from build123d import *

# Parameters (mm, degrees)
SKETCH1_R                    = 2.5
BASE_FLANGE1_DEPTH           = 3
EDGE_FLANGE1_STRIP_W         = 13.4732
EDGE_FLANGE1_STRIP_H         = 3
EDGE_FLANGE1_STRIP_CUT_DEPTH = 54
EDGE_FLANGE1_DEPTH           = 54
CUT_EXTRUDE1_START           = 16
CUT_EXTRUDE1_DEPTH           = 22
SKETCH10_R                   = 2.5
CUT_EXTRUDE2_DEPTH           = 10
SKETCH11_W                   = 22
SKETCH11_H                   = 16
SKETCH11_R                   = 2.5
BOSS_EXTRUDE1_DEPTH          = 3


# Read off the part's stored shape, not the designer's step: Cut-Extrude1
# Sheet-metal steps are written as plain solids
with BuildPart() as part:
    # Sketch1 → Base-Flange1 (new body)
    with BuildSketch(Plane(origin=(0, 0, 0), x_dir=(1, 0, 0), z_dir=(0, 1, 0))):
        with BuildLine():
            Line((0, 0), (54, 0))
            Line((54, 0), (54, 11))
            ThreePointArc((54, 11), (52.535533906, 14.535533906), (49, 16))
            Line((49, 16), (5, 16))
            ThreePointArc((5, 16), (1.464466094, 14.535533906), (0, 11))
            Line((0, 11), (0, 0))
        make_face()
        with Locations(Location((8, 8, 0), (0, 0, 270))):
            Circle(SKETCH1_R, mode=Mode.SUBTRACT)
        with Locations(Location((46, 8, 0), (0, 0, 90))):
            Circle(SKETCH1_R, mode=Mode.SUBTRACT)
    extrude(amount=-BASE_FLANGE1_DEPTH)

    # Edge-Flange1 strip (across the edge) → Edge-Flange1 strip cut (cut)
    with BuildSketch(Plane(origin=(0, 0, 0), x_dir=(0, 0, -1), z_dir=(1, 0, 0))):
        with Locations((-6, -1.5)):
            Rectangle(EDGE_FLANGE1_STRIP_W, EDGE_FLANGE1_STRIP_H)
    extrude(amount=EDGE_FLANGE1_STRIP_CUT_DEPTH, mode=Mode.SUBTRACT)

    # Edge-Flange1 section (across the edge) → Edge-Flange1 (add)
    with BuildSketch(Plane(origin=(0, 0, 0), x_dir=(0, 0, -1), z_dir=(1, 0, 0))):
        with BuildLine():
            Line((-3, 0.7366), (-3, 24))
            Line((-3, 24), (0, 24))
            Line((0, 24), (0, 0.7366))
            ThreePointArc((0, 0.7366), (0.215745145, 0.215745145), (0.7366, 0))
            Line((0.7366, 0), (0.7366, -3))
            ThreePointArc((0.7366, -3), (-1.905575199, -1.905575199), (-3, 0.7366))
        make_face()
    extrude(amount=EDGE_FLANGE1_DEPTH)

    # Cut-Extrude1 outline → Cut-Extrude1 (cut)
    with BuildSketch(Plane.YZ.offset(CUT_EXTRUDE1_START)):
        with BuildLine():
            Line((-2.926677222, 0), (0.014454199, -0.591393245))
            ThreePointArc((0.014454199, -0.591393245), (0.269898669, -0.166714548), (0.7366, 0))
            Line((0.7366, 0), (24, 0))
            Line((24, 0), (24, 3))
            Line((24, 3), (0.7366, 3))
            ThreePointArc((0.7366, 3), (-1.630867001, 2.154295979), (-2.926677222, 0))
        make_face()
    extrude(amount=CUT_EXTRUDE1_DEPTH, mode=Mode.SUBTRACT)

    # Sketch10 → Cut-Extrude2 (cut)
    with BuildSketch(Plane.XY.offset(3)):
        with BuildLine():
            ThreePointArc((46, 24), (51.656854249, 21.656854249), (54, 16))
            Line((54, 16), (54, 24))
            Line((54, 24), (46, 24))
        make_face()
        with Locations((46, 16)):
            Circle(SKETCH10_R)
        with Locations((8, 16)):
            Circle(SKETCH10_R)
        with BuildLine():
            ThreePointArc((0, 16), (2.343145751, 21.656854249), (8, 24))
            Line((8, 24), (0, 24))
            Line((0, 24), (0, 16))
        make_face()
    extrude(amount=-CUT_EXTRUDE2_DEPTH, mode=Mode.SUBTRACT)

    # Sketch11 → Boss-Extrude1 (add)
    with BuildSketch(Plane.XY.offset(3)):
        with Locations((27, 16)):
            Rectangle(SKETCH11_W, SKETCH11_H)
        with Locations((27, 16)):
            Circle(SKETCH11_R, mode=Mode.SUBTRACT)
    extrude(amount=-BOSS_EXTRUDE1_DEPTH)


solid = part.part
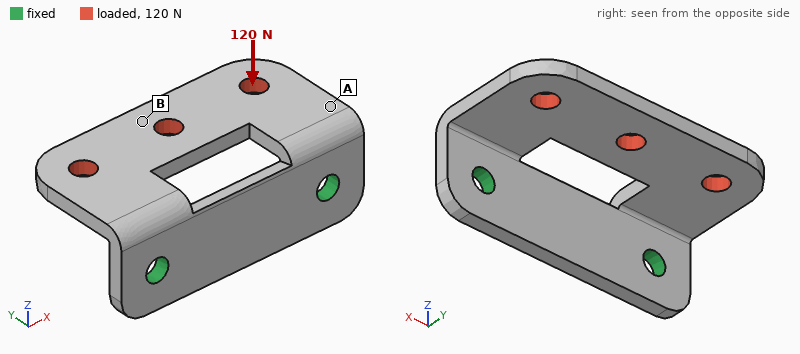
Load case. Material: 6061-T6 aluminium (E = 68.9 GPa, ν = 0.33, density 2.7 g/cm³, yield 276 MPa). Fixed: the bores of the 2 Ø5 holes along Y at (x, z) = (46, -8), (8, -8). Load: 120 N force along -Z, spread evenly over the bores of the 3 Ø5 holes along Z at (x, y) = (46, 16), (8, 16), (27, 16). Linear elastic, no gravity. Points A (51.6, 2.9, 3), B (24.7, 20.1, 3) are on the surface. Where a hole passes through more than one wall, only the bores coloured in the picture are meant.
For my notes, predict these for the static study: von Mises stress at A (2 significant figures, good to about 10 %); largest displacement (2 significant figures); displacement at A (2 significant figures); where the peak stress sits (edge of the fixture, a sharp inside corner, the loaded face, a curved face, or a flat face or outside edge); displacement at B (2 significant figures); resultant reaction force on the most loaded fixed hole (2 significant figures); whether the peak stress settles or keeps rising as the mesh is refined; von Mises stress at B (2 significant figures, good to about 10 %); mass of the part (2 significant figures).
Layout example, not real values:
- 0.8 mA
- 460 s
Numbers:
- 31 MPa
- 0.15 mm
- 0.024 mm
- a sharp inside corner
- 0.13 mm
- 61 N
- keeps rising
- 8.3 MPa
- 15 g
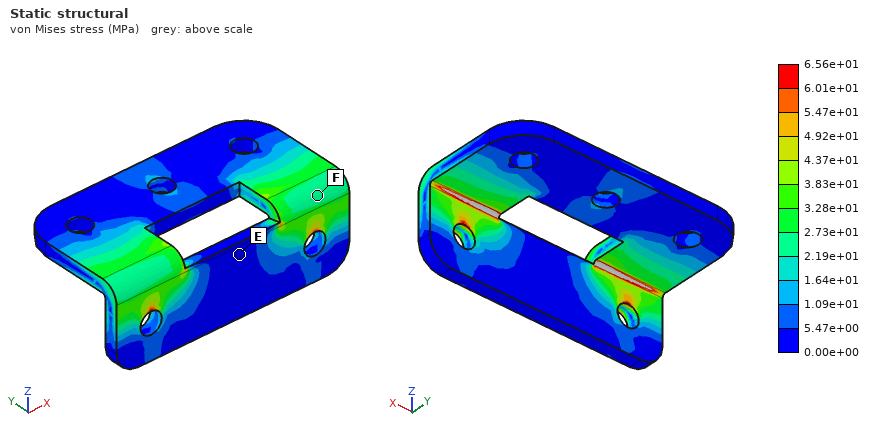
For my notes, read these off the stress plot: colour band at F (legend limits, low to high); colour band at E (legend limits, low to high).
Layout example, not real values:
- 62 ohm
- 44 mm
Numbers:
- 2.19e+01 to 2.73e+01 MPa
- 0.00e+00 to 5.47e+00 MPa
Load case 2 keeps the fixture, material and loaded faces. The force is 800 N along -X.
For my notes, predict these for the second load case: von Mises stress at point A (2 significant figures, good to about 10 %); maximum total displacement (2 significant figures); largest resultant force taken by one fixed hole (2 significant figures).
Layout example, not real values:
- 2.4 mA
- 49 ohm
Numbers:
- 16 MPa
- 73 µm
- 530 N
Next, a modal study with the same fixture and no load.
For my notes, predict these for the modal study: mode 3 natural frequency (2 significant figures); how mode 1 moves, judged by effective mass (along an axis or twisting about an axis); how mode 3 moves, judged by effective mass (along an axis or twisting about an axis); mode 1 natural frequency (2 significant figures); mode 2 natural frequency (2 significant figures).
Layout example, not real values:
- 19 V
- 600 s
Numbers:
- 8700 Hz
- along Z
- along Y
- 2100 Hz
- 4300 Hz
